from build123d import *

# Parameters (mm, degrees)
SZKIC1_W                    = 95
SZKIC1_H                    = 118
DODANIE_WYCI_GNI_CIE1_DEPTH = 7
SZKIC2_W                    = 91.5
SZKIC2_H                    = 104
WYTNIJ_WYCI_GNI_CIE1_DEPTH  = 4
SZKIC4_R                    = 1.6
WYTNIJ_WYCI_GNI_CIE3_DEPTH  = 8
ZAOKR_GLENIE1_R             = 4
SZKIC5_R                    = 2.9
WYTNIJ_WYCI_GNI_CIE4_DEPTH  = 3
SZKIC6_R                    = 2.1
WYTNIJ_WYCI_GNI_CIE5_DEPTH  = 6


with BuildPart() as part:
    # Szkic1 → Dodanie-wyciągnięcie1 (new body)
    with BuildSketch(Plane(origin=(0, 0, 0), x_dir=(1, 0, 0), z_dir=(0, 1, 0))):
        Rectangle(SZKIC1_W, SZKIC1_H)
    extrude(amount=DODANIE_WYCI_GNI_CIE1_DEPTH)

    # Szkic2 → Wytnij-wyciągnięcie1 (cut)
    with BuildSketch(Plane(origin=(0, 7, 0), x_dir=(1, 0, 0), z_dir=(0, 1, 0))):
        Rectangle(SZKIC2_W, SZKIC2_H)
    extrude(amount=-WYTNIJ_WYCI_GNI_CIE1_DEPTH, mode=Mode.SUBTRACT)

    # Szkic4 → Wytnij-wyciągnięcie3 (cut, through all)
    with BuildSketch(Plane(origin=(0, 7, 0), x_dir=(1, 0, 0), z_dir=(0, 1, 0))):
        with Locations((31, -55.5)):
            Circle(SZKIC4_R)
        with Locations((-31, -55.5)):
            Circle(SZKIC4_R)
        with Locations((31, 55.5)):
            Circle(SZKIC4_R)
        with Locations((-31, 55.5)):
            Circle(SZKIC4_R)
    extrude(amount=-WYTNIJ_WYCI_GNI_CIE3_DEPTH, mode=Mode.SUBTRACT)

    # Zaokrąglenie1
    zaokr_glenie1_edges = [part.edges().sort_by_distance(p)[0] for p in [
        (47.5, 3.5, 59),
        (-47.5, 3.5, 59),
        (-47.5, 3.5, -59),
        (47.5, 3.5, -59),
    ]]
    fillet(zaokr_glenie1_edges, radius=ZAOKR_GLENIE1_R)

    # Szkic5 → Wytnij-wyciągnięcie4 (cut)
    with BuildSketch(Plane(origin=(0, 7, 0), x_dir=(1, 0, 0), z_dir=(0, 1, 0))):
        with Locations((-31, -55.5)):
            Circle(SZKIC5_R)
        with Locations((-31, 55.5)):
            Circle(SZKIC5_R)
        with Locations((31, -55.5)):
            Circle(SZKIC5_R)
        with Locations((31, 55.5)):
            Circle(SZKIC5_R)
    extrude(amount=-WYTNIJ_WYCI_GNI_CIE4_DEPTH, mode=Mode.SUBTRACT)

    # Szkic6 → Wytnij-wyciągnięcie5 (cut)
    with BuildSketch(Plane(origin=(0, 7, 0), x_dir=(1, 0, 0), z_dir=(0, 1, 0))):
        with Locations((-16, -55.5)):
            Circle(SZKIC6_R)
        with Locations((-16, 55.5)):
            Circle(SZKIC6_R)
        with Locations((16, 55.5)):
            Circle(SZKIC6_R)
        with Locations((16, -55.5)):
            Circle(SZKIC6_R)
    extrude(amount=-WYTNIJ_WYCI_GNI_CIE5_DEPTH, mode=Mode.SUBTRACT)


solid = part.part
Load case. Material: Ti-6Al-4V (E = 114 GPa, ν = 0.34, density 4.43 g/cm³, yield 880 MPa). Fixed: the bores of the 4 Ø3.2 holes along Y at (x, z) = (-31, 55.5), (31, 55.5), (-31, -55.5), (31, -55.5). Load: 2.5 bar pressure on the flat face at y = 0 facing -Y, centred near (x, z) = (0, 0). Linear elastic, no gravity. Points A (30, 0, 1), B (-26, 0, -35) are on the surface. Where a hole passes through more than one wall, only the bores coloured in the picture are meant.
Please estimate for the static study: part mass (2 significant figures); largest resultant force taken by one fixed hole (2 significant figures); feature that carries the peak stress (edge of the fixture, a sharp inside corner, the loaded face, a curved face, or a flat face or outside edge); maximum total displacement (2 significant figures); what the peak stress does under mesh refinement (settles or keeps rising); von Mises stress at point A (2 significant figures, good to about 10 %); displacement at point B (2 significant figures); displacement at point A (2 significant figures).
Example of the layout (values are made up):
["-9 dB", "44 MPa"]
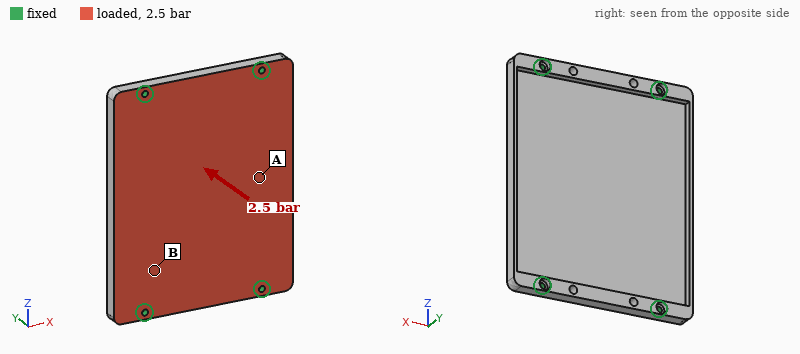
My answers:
["180 g", "740 N", "edge of the fixture", "0.35 mm", "keeps rising", "62 MPa", "0.13 mm", "0.30 mm"]
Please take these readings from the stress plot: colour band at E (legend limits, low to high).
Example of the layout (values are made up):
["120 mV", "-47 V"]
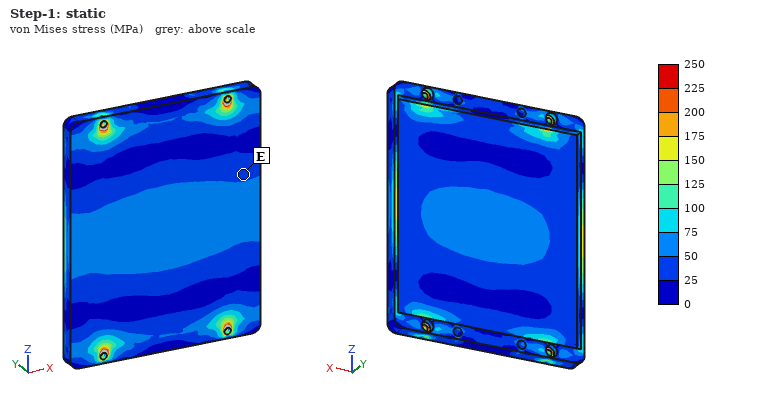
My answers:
["25 to 50 MPa"]
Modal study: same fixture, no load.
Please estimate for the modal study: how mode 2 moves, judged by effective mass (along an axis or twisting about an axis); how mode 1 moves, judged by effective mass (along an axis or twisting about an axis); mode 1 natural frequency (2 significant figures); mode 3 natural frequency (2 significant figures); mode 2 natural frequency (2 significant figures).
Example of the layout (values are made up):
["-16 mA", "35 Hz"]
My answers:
["twisting about Z", "along Y", "1400 Hz", "2800 Hz", "1900 Hz"]
